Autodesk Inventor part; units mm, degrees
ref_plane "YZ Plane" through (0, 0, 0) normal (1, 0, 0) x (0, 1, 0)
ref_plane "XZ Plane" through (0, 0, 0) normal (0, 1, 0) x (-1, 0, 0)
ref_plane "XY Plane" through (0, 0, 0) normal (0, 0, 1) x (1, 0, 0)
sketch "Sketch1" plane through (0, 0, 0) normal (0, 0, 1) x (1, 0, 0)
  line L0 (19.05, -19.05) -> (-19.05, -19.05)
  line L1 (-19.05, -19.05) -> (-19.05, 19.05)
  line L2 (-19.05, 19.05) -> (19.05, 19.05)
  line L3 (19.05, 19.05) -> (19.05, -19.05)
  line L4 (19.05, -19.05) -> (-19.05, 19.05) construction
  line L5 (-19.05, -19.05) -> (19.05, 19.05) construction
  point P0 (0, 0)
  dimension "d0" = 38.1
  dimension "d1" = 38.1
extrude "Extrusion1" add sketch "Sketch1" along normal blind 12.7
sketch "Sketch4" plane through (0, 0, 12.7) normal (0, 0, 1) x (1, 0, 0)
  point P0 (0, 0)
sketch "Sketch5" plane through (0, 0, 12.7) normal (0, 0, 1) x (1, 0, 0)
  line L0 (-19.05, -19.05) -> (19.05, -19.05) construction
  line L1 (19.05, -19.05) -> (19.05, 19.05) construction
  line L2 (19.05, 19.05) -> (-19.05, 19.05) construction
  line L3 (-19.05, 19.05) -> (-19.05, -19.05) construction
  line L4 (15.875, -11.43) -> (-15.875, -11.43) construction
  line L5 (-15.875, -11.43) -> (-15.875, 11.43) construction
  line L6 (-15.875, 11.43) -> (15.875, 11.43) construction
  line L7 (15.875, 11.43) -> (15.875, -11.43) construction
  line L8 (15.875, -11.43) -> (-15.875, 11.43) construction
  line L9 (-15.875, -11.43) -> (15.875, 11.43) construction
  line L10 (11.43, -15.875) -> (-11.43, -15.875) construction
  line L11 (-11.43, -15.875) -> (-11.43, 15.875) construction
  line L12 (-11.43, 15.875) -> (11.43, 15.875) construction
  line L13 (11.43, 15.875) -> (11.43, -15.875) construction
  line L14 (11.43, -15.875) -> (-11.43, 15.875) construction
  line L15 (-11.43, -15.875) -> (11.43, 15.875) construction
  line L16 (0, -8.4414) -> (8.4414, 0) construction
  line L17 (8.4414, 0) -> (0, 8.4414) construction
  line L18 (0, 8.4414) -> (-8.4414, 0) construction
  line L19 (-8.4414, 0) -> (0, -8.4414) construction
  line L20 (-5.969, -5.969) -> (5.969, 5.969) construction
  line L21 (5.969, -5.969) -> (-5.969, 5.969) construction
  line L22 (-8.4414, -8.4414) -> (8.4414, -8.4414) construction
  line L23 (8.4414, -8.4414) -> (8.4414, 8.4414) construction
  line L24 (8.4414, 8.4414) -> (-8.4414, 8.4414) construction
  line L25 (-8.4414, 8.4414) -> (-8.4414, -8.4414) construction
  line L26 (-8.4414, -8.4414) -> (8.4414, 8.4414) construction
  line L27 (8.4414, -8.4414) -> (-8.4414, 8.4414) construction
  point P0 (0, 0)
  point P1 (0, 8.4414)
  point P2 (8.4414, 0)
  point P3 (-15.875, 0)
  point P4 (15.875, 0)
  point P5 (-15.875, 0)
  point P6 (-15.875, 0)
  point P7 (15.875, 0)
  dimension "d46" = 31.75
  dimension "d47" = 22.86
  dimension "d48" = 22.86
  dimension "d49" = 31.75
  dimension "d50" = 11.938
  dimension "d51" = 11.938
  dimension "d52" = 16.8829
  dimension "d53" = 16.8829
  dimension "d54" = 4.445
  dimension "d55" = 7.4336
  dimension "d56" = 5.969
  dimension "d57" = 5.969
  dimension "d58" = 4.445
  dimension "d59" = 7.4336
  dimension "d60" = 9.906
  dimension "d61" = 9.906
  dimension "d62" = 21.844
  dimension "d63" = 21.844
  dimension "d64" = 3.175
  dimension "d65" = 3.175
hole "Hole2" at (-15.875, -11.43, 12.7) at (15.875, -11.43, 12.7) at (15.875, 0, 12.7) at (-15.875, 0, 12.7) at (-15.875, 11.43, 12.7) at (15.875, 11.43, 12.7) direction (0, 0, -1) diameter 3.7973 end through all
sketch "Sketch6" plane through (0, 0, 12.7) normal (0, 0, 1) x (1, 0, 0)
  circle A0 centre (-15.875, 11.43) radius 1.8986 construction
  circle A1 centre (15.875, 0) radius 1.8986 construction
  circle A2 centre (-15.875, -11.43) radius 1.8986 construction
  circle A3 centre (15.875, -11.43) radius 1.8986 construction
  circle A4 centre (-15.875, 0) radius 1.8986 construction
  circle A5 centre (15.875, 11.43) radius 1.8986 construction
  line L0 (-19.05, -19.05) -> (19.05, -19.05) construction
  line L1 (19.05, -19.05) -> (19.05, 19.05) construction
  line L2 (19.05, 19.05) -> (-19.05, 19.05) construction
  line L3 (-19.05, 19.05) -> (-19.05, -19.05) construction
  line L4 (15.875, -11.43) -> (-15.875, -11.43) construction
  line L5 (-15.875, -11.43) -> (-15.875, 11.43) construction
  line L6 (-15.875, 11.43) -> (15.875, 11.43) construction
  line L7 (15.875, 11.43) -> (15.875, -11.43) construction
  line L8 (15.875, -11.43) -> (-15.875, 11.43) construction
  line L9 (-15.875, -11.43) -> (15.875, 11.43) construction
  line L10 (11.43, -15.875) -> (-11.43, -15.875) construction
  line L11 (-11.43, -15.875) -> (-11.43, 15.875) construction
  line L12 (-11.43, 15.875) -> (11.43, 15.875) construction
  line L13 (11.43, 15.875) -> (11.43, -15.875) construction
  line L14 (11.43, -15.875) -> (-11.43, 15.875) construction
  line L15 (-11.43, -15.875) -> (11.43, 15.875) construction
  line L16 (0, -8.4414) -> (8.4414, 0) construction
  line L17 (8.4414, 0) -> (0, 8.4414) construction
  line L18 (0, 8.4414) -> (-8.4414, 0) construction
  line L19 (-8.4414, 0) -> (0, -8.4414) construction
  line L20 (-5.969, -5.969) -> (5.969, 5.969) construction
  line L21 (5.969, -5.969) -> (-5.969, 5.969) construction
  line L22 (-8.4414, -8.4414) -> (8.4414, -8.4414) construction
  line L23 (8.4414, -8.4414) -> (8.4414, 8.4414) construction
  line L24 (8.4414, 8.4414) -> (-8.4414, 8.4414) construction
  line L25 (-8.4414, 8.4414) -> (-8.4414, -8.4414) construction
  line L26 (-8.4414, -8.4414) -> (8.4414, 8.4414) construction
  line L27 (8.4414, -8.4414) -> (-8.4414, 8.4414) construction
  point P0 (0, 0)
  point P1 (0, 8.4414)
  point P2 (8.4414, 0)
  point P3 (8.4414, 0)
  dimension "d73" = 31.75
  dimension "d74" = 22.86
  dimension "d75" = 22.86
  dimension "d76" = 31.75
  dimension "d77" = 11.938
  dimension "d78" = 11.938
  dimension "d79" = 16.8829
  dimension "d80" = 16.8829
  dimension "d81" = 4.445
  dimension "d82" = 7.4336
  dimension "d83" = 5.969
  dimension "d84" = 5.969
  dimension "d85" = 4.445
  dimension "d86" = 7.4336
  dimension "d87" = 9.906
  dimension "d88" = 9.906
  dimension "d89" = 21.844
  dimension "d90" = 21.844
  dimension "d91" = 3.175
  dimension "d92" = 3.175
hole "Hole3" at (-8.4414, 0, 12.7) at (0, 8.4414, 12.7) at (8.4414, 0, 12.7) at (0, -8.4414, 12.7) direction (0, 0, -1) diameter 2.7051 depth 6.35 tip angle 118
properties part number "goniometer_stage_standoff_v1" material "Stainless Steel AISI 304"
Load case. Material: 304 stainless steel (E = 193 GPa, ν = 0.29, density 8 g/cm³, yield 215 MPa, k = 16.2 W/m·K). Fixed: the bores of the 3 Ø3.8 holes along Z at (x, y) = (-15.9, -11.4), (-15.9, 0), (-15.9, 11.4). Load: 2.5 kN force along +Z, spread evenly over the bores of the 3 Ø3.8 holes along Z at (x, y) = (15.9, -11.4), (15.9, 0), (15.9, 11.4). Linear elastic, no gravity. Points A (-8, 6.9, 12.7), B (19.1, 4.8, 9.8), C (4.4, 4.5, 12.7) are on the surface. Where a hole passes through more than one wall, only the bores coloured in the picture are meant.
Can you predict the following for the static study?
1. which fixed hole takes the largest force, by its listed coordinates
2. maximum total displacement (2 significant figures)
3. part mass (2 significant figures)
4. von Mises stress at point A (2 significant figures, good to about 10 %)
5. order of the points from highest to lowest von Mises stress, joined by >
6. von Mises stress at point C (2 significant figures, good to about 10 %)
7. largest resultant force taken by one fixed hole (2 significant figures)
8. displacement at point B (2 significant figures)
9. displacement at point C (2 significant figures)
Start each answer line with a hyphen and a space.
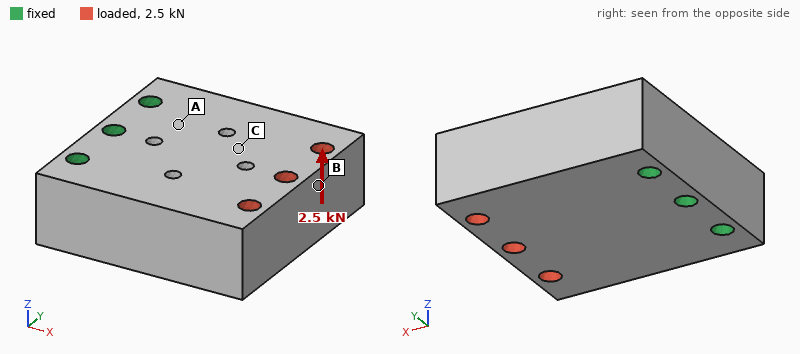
- (-15.9, 0)
- 30 µm
- 140 g
- 53 MPa
- A > C > B
- 31 MPa
- 1.1 kN
- 29 µm
- 14 µm
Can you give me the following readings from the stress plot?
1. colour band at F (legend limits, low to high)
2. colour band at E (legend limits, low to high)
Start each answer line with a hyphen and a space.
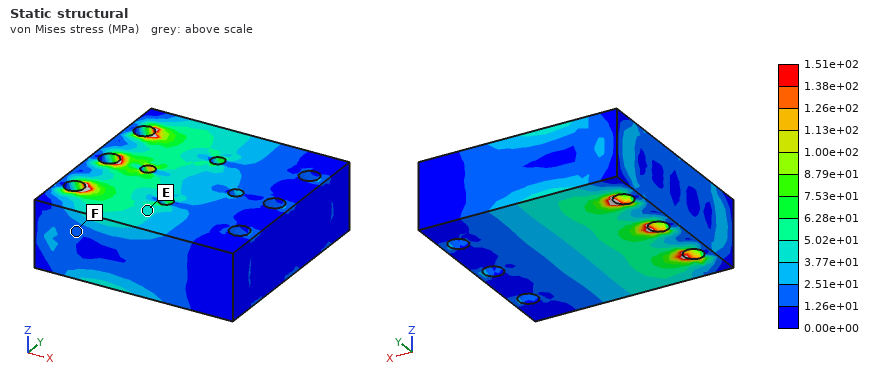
- 1.26e+01 to 2.51e+01 MPa
- 3.77e+01 to 5.02e+01 MPa
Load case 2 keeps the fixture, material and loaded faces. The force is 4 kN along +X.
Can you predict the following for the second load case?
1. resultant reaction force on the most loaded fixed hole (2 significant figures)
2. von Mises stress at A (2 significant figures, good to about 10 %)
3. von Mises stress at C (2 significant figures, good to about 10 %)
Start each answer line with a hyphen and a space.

- 1.4 kN
- 8.0 MPa
- 12 MPa
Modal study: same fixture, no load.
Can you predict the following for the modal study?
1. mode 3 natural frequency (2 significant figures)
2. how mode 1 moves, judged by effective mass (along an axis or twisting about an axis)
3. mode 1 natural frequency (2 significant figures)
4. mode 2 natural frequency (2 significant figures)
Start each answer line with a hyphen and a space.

- 14 kHz
- along Z
- 7700 Hz
- 14 kHz
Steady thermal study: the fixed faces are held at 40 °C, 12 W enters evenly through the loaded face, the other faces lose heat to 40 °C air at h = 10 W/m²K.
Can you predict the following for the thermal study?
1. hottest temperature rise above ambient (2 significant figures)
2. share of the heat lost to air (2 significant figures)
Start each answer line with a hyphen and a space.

- 52 K
- 9.4 %
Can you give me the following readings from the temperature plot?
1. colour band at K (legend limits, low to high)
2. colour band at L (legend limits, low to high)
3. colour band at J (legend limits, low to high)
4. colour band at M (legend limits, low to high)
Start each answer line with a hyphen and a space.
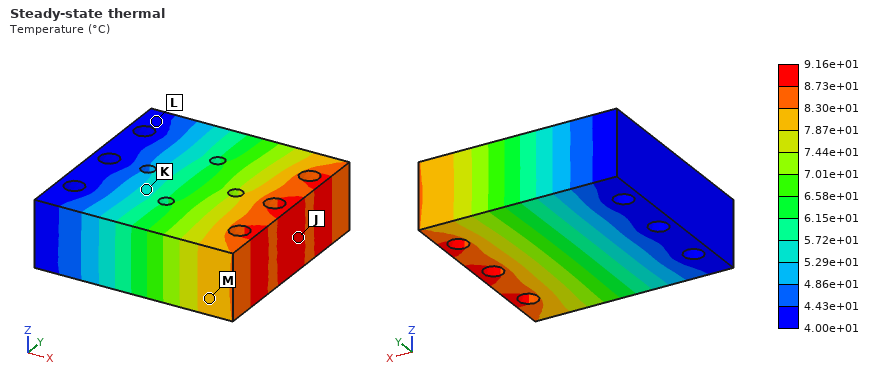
- 5.29e+01 to 5.72e+01 °C
- 4.00e+01 to 4.43e+01 °C
- 8.73e+01 to 9.16e+01 °C
- 7.87e+01 to 8.30e+01 °C
